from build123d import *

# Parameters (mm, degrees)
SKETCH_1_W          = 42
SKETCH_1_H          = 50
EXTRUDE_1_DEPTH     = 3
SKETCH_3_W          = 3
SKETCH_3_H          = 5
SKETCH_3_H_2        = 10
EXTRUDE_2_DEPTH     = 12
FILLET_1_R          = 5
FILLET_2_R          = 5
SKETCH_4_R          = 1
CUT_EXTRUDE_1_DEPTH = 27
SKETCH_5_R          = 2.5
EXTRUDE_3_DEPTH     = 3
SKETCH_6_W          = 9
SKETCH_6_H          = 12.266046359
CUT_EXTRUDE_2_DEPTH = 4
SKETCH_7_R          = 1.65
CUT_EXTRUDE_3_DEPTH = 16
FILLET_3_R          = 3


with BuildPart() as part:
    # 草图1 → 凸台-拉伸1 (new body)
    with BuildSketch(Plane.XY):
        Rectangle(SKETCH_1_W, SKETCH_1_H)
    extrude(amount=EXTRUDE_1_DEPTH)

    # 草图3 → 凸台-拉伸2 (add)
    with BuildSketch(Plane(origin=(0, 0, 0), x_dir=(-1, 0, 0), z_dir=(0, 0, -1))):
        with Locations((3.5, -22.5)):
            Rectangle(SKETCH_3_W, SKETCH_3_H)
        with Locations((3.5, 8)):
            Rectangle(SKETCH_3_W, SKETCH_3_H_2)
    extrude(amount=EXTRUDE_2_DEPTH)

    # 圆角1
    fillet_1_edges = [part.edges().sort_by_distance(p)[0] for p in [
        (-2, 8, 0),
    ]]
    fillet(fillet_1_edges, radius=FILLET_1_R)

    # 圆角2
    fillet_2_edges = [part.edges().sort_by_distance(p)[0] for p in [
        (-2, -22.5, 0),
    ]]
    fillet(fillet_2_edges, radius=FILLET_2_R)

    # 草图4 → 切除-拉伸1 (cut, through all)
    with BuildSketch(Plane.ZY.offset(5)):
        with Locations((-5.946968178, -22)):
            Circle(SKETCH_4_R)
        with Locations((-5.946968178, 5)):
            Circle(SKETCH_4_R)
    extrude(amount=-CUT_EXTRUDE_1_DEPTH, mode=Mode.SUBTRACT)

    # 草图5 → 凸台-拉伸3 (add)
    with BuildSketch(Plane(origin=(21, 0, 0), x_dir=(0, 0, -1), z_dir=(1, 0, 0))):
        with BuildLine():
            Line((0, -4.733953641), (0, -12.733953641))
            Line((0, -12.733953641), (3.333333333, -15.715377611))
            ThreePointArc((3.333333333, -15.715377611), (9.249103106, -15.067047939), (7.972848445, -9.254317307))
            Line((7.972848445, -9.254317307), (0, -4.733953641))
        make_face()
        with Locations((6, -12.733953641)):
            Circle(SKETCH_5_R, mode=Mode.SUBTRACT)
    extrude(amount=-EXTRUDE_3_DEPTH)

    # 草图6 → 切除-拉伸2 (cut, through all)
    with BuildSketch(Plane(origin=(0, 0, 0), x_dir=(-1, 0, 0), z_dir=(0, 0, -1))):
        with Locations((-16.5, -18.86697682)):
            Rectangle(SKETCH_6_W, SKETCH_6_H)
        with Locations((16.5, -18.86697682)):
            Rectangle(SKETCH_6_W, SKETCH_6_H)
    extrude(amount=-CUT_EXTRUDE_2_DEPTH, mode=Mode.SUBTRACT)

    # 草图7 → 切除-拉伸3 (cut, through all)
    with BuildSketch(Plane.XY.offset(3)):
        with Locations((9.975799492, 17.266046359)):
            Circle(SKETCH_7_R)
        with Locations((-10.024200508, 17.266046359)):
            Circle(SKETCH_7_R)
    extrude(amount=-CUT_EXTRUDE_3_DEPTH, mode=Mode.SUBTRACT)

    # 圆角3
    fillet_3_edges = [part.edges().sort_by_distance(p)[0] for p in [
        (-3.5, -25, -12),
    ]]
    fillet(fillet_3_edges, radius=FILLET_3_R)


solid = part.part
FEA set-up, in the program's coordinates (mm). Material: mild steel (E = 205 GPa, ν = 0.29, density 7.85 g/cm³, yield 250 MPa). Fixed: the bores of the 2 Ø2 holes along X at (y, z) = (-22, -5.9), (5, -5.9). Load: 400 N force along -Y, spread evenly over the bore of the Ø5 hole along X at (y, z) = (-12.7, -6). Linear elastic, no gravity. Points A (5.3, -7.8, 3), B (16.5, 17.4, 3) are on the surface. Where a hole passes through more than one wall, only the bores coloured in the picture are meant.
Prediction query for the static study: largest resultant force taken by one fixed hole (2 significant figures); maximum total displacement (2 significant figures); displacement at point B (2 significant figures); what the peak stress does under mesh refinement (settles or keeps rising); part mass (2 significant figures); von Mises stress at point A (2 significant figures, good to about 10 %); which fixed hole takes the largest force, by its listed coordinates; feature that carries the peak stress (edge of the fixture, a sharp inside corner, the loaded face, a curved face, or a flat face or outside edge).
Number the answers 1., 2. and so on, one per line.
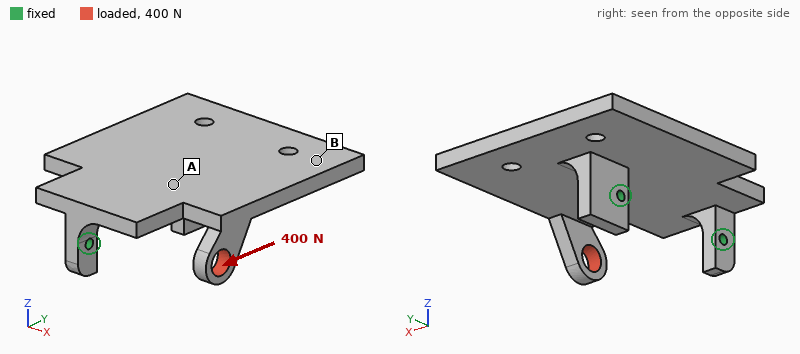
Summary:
1. 400 N
2. 93 µm
3. 38 µm
4. keeps rising
5. 50 g
6. 57 MPa
7. (5, -5.9)
8. edge of the fixture
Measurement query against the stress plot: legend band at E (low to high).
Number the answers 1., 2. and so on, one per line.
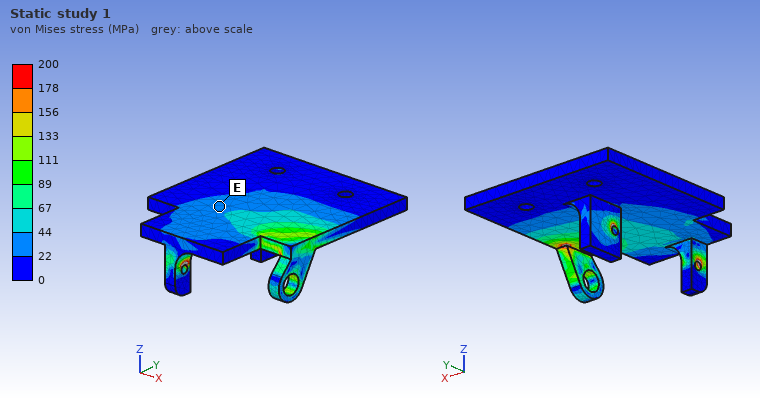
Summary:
1. 22 to 44 MPa
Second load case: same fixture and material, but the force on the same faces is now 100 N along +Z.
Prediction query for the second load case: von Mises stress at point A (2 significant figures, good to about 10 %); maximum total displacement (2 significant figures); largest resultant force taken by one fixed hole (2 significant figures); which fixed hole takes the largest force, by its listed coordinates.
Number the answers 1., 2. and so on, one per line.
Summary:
1. 29 MPa
2. 81 µm
3. 77 N
4. (-22, -5.9)
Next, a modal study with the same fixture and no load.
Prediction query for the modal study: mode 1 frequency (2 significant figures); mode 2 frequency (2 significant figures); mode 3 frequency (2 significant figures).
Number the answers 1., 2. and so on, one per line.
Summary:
1. 1900 Hz
2. 4500 Hz
3. 5300 Hz
